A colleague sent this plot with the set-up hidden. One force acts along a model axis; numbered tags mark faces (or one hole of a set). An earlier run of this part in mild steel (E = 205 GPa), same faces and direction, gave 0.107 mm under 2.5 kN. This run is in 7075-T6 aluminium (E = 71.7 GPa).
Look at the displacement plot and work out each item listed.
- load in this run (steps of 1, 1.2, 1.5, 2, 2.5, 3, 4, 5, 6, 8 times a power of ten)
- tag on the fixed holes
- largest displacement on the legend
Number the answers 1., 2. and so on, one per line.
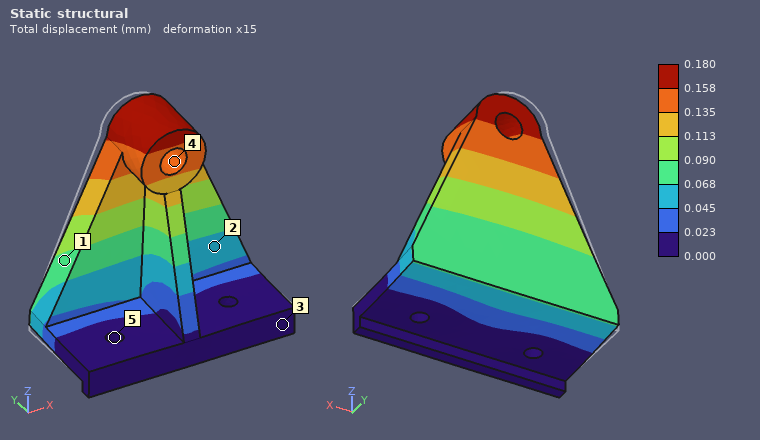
1. 1.5 kN
2. 5
3. 0.180 mm
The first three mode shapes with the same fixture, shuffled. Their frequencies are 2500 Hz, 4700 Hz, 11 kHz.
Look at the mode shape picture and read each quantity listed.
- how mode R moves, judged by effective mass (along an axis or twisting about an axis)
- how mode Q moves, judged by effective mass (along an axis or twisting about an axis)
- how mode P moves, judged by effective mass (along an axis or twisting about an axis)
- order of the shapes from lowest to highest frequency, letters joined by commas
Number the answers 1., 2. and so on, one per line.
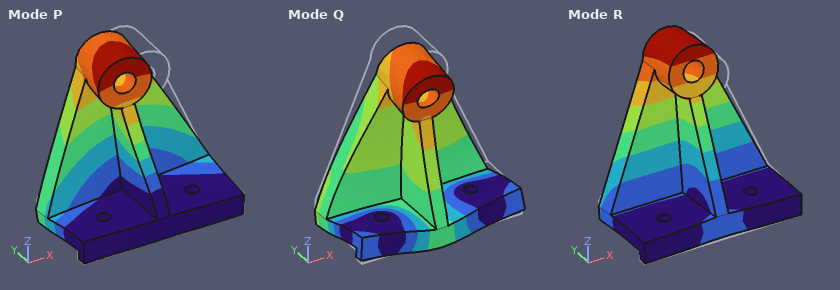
1. along Y
2. along Z
3. along X
4. R, P, Q
